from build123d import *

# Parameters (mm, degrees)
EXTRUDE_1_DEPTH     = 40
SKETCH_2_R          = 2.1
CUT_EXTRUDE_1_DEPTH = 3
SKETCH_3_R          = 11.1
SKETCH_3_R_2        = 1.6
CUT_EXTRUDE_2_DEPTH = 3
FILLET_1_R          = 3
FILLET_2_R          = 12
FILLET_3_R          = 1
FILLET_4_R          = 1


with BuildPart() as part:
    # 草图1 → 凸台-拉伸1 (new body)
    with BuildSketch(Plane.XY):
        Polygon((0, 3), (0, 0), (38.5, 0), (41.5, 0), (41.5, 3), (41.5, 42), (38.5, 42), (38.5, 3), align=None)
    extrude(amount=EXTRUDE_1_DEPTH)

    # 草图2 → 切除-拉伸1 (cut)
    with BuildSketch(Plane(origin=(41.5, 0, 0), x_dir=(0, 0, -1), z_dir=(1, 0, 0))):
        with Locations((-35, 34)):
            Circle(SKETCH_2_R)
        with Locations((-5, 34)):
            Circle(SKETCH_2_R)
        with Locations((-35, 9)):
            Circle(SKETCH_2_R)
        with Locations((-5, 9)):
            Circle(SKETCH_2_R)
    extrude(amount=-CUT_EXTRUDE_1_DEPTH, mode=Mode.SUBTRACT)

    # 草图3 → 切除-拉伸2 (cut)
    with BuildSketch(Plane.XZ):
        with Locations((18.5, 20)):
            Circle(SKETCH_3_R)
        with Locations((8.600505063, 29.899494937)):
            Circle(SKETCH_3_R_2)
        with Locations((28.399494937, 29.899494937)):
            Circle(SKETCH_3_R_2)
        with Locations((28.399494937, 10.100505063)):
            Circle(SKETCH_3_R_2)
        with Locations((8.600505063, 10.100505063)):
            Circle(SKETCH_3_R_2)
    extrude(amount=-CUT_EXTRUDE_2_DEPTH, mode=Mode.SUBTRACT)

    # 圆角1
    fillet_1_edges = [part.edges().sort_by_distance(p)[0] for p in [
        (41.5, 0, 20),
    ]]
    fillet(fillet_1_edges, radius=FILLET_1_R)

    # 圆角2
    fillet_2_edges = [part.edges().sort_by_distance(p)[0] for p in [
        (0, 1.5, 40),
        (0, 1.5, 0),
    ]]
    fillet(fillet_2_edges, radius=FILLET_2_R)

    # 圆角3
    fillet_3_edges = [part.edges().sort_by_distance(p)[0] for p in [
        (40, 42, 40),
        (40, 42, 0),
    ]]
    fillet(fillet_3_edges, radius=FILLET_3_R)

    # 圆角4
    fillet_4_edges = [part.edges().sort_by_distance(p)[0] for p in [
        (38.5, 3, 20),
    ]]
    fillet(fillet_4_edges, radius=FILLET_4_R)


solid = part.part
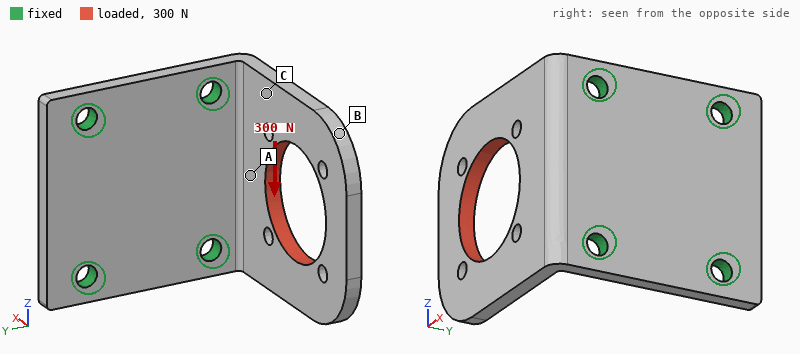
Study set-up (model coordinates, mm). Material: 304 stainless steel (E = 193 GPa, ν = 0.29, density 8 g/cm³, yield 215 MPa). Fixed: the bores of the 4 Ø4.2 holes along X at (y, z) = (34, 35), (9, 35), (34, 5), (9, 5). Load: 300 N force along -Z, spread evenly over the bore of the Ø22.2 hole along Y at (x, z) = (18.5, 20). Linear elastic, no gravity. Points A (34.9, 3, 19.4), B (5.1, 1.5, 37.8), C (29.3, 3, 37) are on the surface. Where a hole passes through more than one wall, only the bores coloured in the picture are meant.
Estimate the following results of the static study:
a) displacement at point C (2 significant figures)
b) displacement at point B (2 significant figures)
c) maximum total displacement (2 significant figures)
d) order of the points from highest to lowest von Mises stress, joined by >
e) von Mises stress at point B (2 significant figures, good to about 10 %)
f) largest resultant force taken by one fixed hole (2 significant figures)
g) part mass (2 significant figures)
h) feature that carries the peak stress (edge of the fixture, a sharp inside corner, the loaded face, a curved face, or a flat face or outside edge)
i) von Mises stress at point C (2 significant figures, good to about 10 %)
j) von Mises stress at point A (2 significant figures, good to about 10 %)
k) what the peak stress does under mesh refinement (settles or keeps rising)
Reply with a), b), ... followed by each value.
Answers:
a) 5.8 µm
b) 13 µm
c) 14 µm
d) A > C > B
e) 4.7 MPa
f) 260 N
g) 64 g
h) edge of the fixture
i) 13 MPa
j) 20 MPa
k) keeps rising
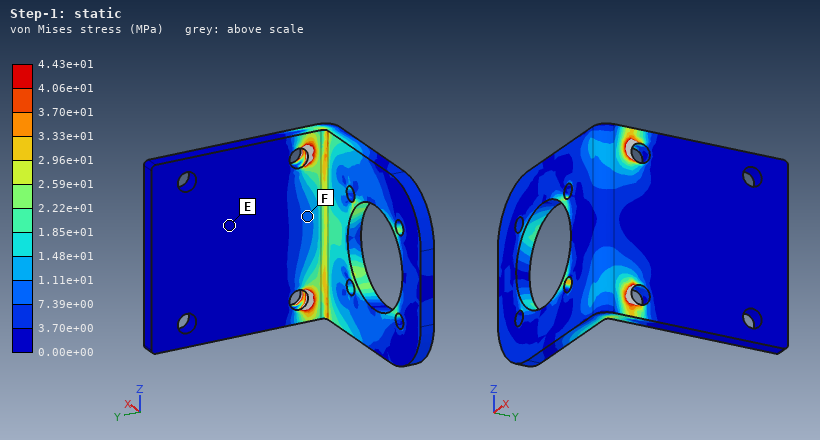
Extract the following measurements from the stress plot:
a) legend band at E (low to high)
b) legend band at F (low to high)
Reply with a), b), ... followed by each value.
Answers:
a) 0.00e+00 to 3.70e+00 MPa
b) 7.39e+00 to 1.11e+01 MPa
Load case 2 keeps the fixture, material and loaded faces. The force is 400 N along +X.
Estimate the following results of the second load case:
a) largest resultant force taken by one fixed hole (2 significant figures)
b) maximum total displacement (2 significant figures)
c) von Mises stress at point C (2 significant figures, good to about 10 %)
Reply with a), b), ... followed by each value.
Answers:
a) 210 N
b) 25 µm
c) 6.1 MPa
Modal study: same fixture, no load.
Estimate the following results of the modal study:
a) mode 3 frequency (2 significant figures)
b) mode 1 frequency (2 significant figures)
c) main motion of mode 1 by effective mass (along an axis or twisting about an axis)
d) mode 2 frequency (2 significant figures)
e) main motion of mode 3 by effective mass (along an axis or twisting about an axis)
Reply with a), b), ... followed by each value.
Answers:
a) 6000 Hz
b) 1300 Hz
c) along Y
d) 3100 Hz
e) along Z
